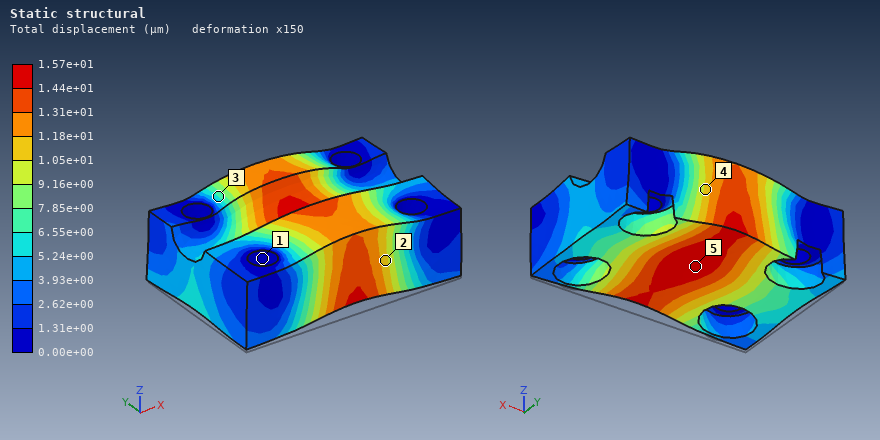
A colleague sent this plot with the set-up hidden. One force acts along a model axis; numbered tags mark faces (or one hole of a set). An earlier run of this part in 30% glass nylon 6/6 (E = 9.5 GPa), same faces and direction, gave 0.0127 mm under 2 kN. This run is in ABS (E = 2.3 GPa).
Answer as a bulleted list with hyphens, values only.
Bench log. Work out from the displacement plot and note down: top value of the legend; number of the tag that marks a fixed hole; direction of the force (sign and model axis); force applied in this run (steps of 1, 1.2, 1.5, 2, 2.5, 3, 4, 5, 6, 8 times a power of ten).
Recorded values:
- 1.57e+01 µm
- 1
- +Z
- 600 N
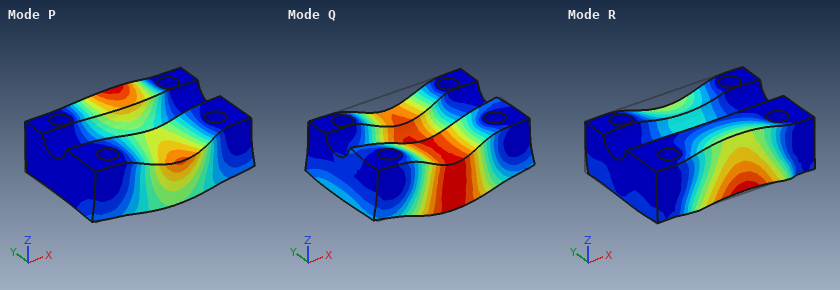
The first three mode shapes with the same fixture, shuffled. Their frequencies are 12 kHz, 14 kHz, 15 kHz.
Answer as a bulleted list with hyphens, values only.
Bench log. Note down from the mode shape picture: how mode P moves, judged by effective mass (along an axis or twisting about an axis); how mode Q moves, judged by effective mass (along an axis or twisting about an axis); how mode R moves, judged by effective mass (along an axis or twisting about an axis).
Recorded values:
- along Y
- along Z
- along Y
